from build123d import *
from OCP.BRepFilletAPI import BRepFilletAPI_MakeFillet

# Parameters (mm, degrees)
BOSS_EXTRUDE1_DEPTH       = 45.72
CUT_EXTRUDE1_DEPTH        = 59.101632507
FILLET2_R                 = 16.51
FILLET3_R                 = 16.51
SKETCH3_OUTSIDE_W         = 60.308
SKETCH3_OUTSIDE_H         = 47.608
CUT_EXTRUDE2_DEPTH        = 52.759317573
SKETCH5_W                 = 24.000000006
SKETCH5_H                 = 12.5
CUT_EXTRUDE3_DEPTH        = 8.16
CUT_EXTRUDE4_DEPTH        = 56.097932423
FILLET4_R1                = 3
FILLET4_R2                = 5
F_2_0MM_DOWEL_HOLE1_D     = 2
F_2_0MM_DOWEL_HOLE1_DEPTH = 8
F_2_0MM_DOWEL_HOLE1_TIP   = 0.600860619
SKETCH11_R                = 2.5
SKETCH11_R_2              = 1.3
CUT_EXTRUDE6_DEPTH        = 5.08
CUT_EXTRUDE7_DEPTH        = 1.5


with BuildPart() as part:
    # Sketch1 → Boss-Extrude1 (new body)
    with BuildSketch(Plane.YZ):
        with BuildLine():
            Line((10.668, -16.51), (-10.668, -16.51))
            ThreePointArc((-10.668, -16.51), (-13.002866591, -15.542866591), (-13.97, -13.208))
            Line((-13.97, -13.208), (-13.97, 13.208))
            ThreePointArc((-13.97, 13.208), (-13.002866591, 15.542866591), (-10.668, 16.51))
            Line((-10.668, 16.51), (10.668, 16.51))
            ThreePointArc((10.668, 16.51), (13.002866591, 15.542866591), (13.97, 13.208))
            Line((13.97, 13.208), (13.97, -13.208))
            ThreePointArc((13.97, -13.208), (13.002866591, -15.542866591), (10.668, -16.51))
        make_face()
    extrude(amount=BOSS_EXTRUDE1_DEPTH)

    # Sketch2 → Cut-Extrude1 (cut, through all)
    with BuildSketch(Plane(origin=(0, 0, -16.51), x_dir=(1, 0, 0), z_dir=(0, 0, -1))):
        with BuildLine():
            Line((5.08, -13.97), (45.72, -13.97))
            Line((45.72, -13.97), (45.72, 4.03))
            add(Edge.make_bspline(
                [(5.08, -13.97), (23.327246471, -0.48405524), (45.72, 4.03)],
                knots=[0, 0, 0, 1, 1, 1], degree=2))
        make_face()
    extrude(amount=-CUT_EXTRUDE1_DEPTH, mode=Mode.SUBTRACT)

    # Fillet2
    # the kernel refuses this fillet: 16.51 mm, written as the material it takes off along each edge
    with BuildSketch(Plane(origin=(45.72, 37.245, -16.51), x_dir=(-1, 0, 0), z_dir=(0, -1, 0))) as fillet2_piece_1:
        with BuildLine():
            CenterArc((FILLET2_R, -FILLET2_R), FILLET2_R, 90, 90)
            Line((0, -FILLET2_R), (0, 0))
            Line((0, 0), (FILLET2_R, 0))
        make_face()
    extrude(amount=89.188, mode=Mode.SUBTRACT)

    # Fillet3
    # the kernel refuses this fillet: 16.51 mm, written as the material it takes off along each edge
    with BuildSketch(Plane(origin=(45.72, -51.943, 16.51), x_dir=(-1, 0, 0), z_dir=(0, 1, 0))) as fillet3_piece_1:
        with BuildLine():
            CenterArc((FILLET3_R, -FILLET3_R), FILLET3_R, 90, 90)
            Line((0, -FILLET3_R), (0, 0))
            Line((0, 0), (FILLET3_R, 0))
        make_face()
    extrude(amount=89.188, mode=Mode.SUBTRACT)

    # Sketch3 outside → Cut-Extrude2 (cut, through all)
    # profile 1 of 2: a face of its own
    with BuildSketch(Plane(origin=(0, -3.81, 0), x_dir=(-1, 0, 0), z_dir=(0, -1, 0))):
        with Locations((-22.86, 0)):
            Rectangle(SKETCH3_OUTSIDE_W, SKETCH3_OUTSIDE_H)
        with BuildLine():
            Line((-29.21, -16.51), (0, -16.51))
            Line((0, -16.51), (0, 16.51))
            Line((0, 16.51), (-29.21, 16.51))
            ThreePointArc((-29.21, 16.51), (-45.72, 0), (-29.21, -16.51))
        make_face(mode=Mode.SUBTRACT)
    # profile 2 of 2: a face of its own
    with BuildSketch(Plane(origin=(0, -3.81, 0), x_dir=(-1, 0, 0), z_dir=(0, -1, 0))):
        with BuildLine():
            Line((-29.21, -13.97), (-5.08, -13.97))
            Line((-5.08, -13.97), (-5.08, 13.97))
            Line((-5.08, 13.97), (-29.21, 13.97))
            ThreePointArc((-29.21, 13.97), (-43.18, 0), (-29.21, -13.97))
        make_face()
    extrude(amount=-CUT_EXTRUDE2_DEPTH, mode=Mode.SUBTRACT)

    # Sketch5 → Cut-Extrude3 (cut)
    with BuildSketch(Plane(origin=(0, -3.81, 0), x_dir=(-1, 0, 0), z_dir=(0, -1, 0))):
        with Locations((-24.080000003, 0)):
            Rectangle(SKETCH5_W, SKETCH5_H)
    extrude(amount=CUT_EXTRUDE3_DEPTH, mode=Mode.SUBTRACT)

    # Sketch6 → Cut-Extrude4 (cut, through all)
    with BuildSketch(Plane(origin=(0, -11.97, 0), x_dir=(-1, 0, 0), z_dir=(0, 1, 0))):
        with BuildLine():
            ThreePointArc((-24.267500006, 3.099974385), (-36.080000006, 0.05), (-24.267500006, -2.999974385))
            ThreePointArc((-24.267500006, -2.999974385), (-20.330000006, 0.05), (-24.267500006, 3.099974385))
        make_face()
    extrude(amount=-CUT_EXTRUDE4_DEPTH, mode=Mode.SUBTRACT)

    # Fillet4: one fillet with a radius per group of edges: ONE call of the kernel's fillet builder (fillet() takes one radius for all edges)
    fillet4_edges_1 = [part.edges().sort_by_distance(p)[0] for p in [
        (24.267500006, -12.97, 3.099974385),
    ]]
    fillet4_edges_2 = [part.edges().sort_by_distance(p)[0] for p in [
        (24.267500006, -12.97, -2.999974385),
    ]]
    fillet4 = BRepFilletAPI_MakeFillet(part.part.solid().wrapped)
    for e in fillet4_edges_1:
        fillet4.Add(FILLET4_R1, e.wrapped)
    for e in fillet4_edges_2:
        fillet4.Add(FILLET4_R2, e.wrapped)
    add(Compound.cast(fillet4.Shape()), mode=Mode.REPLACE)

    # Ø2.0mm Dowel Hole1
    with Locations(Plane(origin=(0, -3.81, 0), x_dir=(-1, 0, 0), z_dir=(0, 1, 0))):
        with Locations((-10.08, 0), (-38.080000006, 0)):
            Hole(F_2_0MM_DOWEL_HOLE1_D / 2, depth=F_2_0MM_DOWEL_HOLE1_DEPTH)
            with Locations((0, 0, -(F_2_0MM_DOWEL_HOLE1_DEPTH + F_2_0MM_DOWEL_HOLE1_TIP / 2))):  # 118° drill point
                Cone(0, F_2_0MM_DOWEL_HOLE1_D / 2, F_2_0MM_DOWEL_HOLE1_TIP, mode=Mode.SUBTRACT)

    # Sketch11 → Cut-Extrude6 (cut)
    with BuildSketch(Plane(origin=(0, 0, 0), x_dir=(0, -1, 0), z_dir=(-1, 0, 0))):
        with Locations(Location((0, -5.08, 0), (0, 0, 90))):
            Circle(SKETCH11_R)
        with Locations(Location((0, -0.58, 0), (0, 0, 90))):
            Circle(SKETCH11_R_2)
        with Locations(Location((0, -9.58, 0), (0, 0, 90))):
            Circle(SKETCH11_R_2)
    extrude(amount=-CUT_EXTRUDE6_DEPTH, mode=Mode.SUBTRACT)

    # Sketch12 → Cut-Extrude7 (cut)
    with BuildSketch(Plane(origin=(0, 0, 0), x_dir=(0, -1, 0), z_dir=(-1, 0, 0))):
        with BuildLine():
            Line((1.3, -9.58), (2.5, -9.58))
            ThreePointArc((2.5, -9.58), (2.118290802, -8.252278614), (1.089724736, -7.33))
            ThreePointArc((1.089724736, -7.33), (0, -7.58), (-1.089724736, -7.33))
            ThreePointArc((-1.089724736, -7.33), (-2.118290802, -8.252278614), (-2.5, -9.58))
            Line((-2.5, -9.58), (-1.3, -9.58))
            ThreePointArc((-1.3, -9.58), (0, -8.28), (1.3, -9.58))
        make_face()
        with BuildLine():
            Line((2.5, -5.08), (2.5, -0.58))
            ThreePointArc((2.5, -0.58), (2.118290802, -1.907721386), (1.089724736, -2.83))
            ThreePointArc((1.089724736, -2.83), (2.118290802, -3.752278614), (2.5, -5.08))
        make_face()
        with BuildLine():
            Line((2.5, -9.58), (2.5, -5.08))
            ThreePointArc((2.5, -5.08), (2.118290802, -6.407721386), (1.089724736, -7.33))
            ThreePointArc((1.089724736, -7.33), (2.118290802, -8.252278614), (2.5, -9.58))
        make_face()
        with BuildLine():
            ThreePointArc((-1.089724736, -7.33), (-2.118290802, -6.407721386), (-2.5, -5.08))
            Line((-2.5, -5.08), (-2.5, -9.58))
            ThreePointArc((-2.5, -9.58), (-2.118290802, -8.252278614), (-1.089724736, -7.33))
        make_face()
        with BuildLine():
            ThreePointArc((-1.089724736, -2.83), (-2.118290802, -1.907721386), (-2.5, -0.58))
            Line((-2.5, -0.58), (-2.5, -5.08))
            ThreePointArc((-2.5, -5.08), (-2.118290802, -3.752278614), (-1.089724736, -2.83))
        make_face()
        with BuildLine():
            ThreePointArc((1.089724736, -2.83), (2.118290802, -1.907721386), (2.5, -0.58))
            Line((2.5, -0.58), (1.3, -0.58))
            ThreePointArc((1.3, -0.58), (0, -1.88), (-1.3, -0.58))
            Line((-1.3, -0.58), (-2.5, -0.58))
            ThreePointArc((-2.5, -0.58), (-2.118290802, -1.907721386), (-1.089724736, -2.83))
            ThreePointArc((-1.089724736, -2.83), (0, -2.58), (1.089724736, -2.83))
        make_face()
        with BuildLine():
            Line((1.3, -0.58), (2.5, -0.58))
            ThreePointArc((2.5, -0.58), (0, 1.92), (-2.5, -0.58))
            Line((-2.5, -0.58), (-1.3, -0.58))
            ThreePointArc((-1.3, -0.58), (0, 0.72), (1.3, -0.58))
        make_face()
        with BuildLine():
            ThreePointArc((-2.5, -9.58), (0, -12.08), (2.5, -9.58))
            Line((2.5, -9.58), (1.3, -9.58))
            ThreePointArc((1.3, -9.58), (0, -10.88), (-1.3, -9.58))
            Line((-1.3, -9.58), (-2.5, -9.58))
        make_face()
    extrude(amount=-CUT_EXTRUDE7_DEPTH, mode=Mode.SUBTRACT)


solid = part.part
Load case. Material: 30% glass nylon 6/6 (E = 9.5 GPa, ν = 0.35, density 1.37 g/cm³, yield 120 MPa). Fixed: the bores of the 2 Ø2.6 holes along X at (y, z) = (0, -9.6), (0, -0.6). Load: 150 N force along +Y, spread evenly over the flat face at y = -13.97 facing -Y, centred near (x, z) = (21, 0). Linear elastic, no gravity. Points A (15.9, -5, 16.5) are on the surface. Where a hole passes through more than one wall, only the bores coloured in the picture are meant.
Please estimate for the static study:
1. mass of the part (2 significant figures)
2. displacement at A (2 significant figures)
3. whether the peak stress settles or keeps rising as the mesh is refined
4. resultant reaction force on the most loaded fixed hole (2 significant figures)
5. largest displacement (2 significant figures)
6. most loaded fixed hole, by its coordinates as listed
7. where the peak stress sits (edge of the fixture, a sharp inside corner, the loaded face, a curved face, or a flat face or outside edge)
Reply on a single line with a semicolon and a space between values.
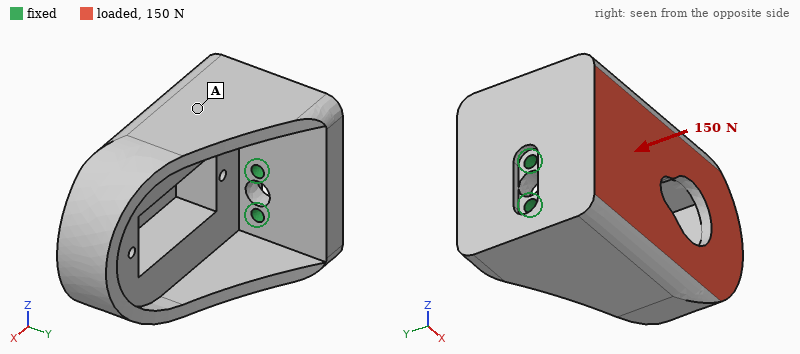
21 g; 0.11 mm; keeps rising; 150 N; 0.34 mm; (0, -0.6); edge of the fixture
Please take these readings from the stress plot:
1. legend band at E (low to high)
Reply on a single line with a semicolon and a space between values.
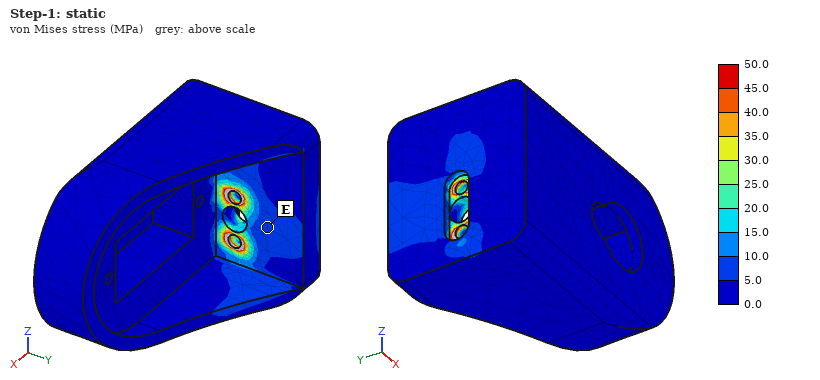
5.0 to 10.0 MPa
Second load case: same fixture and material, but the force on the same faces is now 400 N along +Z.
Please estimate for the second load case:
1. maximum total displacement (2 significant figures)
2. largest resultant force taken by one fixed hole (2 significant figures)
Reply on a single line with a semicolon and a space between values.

0.29 mm; 770 N
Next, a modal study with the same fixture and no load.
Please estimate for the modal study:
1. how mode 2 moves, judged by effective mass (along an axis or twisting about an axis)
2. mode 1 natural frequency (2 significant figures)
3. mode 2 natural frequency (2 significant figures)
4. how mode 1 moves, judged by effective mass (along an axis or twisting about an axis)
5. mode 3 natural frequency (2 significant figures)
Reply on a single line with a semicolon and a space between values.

along Z; 990 Hz; 1600 Hz; along Y; 3700 Hz
